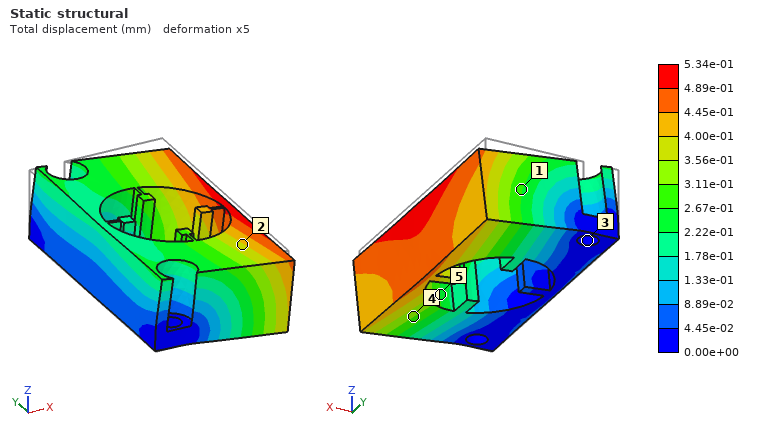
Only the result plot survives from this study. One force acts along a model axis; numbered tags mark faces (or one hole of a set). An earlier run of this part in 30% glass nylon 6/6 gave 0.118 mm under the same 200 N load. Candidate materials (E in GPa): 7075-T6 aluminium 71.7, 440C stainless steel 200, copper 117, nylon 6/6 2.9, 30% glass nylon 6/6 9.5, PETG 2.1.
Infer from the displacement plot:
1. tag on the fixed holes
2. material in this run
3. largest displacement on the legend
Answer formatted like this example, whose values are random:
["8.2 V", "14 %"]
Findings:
["3", "PETG", "5.34e-01 mm"]
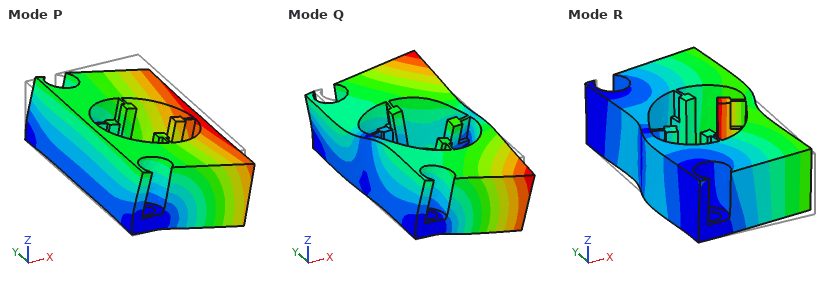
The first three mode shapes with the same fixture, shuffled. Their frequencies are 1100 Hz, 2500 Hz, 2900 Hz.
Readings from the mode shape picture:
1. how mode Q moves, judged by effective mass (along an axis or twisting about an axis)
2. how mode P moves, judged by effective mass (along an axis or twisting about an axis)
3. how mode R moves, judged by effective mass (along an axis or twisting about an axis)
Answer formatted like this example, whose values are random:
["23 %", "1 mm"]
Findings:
["twisting about X", "along Z", "along Y"]
